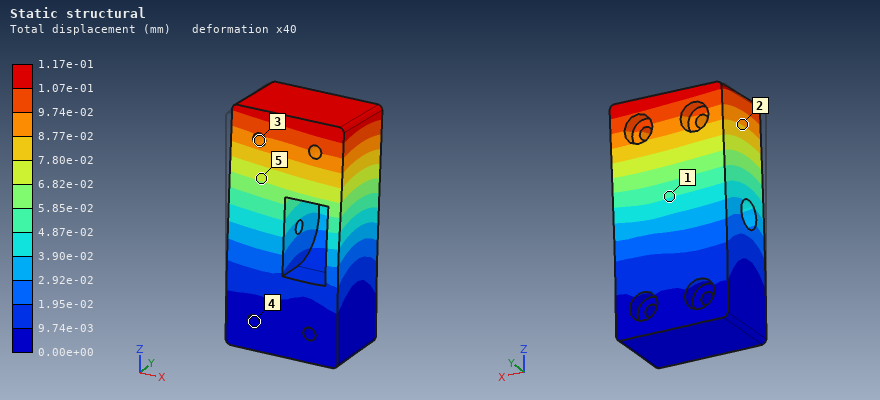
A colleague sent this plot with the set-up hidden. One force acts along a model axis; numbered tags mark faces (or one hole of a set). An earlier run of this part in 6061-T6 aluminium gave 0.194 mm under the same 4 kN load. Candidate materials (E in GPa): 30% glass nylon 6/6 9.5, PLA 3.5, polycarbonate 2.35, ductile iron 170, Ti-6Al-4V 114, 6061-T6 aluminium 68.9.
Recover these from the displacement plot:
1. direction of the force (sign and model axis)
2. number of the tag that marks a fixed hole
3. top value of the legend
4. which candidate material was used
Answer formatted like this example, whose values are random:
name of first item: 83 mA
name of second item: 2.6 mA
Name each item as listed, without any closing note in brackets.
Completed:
direction of the force: +Y
number of the tag that marks a fixed hole: 4
top value of the legend: 1.17e-01 mm
which candidate material was used: Ti-6Al-4V
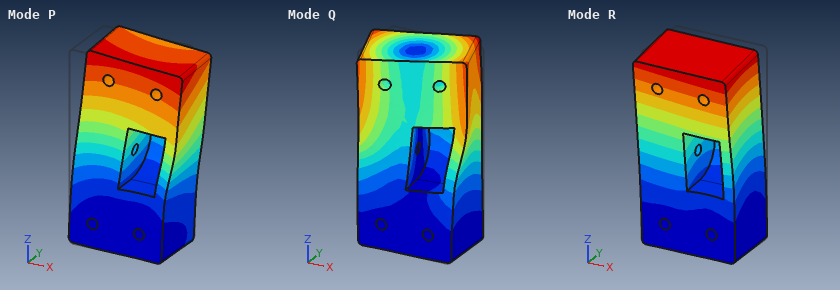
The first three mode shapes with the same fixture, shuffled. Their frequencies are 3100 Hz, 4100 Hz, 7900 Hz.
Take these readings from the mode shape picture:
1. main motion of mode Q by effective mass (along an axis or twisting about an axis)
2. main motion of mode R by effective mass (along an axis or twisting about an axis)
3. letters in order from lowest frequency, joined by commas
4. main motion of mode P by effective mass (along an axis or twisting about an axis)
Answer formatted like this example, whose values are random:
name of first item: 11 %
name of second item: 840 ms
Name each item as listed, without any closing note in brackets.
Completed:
main motion of mode Q by effective mass: twisting about Z
main motion of mode R by effective mass: along Y
letters in order from lowest frequency, joined by commas: R, P, Q
main motion of mode P by effective mass: along X
